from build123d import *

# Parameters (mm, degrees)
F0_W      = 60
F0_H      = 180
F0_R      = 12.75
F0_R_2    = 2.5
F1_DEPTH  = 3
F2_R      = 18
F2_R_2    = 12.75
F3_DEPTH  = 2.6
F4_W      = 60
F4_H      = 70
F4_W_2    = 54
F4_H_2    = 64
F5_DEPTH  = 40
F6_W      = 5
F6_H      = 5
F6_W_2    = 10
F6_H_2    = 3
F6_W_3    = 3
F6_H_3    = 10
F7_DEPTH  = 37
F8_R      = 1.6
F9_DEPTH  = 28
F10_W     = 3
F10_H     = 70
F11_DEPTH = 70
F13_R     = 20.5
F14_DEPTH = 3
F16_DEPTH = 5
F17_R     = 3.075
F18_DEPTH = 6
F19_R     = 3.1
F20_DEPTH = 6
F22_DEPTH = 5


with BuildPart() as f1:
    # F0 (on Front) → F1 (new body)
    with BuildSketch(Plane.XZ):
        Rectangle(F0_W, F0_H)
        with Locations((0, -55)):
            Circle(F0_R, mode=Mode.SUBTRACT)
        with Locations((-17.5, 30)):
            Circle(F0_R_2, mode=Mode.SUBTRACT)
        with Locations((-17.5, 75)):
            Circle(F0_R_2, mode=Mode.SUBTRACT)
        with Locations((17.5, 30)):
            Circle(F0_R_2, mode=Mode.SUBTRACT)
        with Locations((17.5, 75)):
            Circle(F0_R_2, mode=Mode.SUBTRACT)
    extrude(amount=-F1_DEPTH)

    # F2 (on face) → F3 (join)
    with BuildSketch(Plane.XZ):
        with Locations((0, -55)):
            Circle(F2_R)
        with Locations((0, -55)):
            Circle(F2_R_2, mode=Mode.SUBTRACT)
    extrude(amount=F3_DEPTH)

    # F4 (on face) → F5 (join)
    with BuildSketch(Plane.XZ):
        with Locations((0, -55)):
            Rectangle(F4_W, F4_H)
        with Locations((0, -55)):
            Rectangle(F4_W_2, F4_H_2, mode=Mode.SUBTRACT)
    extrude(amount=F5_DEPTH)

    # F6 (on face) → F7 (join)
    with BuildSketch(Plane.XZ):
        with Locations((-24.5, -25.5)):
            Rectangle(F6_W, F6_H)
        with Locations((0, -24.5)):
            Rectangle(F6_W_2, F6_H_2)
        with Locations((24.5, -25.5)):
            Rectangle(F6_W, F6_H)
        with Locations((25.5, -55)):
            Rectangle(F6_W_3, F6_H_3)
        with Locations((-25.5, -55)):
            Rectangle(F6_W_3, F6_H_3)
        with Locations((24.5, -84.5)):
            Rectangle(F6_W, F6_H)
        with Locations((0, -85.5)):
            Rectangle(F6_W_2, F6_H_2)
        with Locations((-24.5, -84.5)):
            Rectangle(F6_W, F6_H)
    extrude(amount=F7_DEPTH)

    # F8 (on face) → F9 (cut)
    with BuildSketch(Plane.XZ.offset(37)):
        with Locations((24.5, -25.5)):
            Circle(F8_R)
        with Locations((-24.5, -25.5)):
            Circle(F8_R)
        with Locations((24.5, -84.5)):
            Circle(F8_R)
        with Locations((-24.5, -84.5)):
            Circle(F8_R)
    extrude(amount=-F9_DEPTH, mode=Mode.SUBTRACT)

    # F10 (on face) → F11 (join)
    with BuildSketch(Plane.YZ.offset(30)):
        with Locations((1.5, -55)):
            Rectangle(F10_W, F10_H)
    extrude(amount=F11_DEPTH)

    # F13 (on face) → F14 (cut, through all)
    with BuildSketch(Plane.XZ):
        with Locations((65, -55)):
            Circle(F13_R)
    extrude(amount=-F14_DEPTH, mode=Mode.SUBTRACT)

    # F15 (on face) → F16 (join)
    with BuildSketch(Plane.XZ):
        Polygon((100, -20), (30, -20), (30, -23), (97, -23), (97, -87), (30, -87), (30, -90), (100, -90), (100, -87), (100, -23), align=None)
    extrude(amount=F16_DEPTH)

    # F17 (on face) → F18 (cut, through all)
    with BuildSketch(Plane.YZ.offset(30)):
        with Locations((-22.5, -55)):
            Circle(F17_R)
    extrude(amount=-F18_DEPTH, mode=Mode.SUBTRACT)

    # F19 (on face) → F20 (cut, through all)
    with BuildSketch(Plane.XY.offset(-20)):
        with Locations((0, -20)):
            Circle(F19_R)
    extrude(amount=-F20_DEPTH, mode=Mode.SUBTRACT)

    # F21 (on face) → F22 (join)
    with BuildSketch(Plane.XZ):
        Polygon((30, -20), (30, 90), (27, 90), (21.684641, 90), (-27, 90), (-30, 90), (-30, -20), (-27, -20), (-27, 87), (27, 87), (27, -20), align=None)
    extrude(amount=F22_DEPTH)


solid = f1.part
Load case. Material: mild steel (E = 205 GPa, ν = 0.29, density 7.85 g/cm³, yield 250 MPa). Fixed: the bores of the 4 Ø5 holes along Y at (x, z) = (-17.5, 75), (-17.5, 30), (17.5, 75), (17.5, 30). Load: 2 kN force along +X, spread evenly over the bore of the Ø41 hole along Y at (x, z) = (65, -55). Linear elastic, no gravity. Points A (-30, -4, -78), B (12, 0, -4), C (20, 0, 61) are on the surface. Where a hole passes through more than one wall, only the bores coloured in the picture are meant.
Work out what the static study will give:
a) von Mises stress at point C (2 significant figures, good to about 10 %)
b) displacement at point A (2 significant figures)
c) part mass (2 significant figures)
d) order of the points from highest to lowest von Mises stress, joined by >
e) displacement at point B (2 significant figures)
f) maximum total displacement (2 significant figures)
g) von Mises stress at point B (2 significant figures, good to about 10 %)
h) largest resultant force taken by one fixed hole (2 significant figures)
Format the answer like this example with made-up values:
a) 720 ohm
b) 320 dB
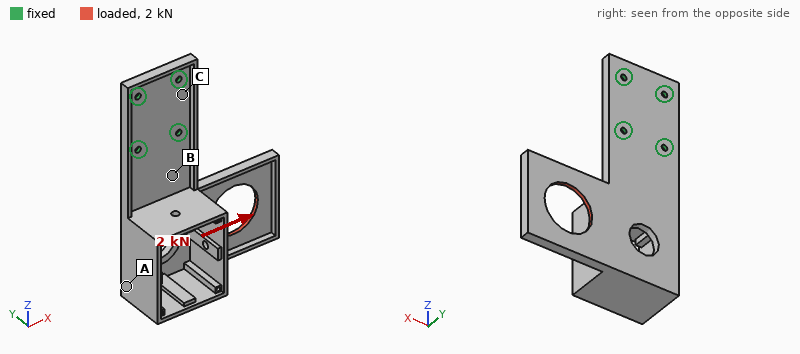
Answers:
a) 14 MPa
b) 66 µm
c) 680 g
d) B > C > A
e) 15 µm
f) 99 µm
g) 29 MPa
h) 3.5 kN
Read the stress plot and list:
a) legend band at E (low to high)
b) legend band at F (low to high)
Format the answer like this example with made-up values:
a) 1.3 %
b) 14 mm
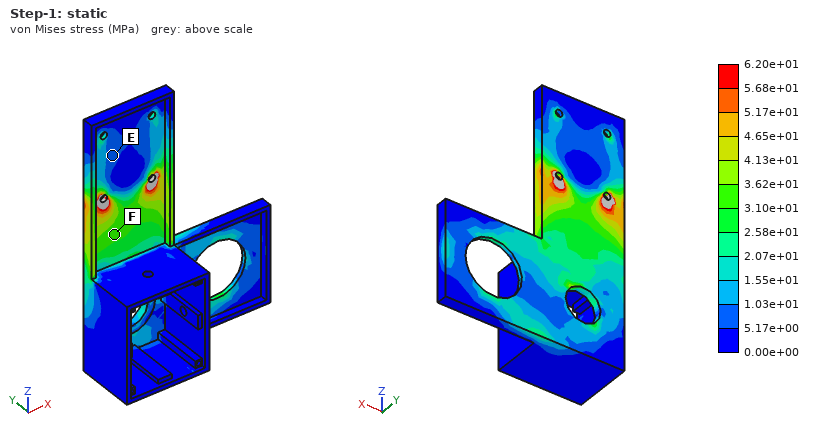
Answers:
a) 5.17e+00 to 1.03e+01 MPa
b) 3.10e+01 to 3.62e+01 MPa
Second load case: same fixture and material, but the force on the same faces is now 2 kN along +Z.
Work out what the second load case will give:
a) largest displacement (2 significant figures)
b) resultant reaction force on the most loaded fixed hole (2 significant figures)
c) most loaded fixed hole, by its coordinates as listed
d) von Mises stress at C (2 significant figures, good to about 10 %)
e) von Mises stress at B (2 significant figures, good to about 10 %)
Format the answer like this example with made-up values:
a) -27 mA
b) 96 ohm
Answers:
a) 0.13 mm
b) 3.3 kN
c) (17.5, 30)
d) 12 MPa
e) 25 MPa
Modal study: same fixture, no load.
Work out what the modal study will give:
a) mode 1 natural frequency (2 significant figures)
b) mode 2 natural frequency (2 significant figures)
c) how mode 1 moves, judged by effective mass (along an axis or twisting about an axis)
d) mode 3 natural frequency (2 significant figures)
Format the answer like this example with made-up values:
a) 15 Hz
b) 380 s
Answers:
a) 140 Hz
b) 310 Hz
c) along Y
d) 1000 Hz
